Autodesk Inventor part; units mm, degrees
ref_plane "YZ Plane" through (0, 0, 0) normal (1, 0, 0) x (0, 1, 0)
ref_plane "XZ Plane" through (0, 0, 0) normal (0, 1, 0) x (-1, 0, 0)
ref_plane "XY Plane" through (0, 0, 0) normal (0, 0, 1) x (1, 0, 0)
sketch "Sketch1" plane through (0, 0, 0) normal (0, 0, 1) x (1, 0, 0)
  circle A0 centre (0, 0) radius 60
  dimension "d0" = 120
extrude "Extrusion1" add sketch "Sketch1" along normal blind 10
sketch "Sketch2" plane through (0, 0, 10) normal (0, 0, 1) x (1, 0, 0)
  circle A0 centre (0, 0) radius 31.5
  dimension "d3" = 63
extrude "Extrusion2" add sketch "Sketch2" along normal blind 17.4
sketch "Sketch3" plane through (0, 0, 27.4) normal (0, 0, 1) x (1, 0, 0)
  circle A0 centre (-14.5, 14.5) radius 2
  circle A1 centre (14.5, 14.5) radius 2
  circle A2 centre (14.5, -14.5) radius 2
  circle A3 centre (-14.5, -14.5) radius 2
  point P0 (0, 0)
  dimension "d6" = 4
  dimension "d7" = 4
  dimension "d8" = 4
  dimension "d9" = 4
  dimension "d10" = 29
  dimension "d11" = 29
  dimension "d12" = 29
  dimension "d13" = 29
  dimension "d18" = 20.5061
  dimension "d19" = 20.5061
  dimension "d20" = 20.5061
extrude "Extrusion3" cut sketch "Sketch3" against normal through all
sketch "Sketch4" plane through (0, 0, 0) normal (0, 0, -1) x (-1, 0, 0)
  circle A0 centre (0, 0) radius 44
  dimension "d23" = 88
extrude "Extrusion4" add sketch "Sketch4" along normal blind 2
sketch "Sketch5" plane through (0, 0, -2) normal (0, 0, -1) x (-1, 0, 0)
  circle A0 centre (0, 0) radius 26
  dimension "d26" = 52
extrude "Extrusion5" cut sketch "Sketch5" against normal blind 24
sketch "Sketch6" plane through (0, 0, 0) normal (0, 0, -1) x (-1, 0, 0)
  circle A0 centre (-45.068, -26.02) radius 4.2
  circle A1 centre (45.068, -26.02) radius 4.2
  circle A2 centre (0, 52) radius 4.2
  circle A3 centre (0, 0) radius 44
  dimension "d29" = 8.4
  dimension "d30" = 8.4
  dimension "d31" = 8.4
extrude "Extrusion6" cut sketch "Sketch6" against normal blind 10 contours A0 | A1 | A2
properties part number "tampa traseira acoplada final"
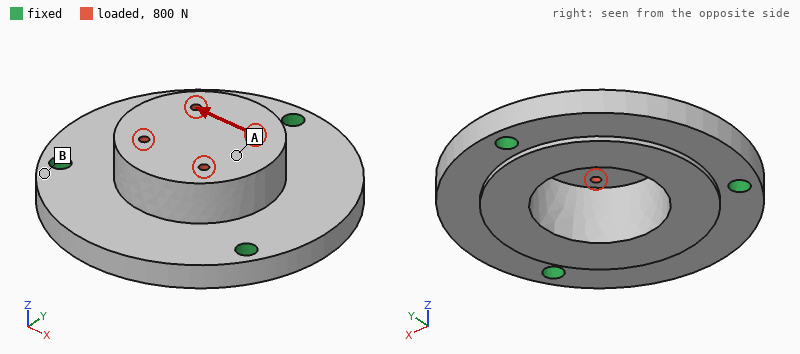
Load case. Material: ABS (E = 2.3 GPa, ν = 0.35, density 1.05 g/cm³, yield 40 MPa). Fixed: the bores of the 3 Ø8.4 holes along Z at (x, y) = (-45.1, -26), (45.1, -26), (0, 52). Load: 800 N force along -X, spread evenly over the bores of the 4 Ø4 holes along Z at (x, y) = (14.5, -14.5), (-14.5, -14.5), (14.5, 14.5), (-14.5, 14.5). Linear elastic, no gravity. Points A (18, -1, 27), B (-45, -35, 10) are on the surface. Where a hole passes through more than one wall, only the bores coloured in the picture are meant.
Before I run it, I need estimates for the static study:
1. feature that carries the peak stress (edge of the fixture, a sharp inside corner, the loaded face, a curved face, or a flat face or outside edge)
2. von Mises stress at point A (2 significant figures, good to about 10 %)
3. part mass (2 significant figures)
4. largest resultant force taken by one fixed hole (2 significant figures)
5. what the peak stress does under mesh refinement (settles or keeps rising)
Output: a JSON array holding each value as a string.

["edge of the fixture", "1.5 MPa", "130 g", "320 N", "keeps rising"]
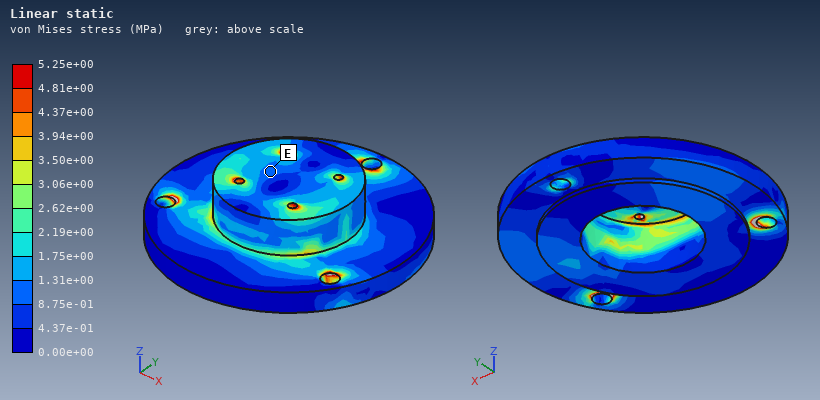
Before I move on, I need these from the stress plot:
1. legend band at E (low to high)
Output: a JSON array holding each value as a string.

["8.75e-01 to 1.31e+00 MPa"]
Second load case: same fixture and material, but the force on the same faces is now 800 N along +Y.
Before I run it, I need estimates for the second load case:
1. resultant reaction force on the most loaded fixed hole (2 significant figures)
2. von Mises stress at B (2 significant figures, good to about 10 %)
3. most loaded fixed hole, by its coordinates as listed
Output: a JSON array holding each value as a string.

["330 N", "1.6 MPa", "(0, 52)"]
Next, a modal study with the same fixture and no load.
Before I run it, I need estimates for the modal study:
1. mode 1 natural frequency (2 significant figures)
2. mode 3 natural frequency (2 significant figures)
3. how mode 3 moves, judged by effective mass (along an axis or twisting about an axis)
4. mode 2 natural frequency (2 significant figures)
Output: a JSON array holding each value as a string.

["1500 Hz", "1600 Hz", "along Z", "1500 Hz"]
